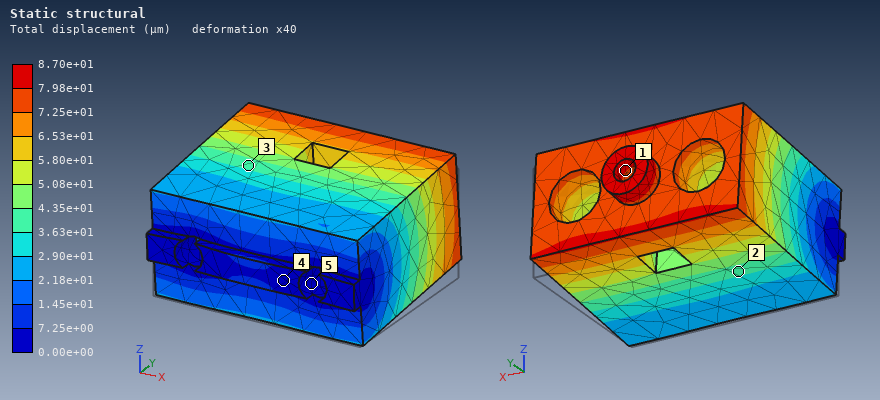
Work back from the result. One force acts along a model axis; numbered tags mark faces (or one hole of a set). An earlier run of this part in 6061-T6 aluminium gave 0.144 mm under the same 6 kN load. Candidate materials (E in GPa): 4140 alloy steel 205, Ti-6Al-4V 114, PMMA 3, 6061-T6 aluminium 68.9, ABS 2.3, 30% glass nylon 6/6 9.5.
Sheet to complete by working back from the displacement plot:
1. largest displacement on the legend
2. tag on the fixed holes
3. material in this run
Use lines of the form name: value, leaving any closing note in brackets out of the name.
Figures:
largest displacement on the legend: 8.70e+01 µm
tag on the fixed holes: 5
material in this run: Ti-6Al-4V
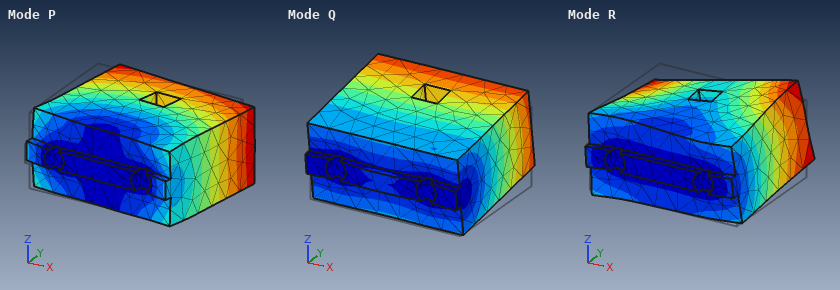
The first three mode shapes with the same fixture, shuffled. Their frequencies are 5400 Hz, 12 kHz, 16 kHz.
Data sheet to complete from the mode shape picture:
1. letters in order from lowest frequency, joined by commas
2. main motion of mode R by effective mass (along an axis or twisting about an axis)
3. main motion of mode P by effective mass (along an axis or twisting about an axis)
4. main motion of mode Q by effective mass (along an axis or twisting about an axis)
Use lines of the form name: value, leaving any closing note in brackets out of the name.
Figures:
letters in order from lowest frequency, joined by commas: Q, P, R
main motion of mode R by effective mass: twisting about Y
main motion of mode P by effective mass: along X
main motion of mode Q by effective mass: along Z
